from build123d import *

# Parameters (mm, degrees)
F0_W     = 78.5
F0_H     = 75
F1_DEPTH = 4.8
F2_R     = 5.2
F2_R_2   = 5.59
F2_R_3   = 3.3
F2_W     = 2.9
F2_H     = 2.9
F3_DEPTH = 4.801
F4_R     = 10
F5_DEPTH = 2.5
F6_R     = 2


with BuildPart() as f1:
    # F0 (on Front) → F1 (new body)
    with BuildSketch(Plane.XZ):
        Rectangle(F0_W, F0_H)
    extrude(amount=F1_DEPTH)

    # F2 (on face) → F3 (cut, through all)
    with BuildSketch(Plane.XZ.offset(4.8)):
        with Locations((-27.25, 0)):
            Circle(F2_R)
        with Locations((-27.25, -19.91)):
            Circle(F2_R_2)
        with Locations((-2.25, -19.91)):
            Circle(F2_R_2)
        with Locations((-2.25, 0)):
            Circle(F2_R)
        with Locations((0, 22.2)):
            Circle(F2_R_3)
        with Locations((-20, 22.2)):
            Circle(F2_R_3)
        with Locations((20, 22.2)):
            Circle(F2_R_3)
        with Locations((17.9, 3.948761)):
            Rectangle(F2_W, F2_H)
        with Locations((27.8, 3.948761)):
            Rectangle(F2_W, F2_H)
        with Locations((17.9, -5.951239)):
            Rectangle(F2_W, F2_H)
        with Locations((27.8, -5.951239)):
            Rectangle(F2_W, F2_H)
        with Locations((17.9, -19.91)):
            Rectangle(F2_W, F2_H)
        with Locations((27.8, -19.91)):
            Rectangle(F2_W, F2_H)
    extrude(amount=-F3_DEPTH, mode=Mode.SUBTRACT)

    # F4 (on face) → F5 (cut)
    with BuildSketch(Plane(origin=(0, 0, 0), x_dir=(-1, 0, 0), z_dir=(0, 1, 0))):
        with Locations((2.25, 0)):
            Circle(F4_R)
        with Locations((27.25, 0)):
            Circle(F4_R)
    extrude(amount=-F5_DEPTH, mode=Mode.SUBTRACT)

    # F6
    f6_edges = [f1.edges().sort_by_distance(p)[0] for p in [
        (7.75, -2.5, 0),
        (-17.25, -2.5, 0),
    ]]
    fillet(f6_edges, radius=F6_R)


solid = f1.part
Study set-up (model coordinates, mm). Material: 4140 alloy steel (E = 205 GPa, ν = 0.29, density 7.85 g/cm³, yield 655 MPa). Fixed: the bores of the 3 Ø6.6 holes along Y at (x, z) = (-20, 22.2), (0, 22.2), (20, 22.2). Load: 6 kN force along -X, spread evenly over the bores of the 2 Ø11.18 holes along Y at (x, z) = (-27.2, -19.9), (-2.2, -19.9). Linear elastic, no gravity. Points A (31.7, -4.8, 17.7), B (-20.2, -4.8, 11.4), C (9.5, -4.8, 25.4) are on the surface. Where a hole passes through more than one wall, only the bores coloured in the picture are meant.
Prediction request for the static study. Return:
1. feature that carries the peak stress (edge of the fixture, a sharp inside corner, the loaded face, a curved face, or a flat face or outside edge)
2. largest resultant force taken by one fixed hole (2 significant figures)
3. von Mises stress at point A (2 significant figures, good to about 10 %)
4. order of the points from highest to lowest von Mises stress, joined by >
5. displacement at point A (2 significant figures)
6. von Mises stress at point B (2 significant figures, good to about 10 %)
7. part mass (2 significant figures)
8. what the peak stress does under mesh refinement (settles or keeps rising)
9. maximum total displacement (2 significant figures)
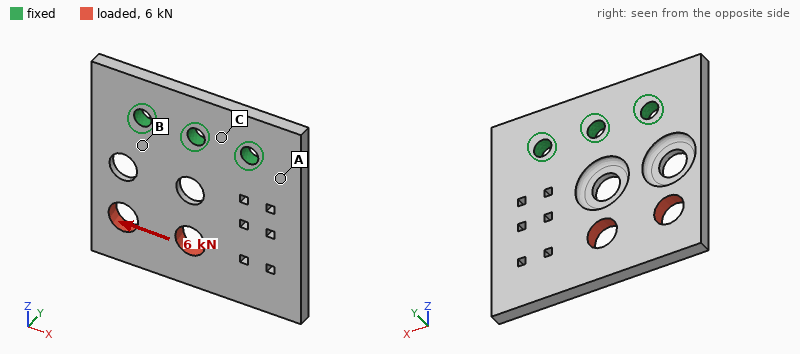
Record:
edge of the fixture
6.0 kN
37 MPa
B > A > C
7.7 µm
77 MPa
190 g
keeps rising
46 µm
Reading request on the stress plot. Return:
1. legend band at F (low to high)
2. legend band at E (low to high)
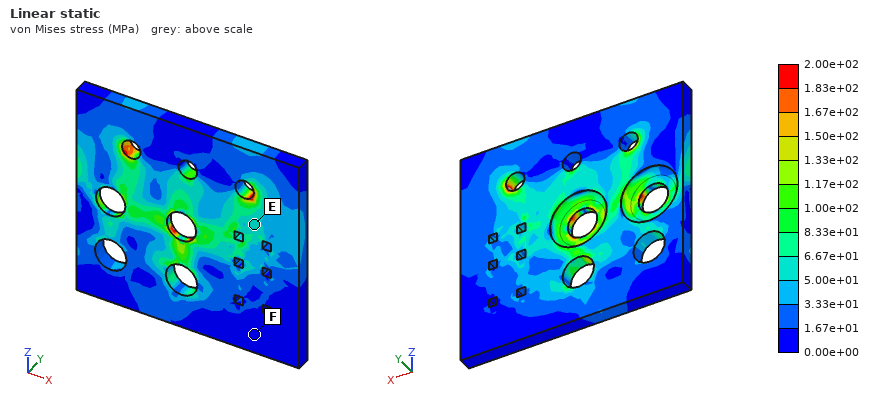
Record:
0.00e+00 to 1.67e+01 MPa
5.00e+01 to 6.67e+01 MPa
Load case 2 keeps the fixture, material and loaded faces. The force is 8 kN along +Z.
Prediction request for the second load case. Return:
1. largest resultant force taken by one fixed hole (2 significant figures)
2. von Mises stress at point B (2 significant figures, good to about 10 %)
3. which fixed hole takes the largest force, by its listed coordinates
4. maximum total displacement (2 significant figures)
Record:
5.8 kN
74 MPa
(-20, 22.2)
57 µm
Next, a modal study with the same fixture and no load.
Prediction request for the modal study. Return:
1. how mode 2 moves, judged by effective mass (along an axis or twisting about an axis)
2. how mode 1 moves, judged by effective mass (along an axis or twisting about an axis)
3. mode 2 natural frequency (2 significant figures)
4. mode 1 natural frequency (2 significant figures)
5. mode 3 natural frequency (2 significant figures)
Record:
twisting about Z
along Y
2000 Hz
1000 Hz
4800 Hz
